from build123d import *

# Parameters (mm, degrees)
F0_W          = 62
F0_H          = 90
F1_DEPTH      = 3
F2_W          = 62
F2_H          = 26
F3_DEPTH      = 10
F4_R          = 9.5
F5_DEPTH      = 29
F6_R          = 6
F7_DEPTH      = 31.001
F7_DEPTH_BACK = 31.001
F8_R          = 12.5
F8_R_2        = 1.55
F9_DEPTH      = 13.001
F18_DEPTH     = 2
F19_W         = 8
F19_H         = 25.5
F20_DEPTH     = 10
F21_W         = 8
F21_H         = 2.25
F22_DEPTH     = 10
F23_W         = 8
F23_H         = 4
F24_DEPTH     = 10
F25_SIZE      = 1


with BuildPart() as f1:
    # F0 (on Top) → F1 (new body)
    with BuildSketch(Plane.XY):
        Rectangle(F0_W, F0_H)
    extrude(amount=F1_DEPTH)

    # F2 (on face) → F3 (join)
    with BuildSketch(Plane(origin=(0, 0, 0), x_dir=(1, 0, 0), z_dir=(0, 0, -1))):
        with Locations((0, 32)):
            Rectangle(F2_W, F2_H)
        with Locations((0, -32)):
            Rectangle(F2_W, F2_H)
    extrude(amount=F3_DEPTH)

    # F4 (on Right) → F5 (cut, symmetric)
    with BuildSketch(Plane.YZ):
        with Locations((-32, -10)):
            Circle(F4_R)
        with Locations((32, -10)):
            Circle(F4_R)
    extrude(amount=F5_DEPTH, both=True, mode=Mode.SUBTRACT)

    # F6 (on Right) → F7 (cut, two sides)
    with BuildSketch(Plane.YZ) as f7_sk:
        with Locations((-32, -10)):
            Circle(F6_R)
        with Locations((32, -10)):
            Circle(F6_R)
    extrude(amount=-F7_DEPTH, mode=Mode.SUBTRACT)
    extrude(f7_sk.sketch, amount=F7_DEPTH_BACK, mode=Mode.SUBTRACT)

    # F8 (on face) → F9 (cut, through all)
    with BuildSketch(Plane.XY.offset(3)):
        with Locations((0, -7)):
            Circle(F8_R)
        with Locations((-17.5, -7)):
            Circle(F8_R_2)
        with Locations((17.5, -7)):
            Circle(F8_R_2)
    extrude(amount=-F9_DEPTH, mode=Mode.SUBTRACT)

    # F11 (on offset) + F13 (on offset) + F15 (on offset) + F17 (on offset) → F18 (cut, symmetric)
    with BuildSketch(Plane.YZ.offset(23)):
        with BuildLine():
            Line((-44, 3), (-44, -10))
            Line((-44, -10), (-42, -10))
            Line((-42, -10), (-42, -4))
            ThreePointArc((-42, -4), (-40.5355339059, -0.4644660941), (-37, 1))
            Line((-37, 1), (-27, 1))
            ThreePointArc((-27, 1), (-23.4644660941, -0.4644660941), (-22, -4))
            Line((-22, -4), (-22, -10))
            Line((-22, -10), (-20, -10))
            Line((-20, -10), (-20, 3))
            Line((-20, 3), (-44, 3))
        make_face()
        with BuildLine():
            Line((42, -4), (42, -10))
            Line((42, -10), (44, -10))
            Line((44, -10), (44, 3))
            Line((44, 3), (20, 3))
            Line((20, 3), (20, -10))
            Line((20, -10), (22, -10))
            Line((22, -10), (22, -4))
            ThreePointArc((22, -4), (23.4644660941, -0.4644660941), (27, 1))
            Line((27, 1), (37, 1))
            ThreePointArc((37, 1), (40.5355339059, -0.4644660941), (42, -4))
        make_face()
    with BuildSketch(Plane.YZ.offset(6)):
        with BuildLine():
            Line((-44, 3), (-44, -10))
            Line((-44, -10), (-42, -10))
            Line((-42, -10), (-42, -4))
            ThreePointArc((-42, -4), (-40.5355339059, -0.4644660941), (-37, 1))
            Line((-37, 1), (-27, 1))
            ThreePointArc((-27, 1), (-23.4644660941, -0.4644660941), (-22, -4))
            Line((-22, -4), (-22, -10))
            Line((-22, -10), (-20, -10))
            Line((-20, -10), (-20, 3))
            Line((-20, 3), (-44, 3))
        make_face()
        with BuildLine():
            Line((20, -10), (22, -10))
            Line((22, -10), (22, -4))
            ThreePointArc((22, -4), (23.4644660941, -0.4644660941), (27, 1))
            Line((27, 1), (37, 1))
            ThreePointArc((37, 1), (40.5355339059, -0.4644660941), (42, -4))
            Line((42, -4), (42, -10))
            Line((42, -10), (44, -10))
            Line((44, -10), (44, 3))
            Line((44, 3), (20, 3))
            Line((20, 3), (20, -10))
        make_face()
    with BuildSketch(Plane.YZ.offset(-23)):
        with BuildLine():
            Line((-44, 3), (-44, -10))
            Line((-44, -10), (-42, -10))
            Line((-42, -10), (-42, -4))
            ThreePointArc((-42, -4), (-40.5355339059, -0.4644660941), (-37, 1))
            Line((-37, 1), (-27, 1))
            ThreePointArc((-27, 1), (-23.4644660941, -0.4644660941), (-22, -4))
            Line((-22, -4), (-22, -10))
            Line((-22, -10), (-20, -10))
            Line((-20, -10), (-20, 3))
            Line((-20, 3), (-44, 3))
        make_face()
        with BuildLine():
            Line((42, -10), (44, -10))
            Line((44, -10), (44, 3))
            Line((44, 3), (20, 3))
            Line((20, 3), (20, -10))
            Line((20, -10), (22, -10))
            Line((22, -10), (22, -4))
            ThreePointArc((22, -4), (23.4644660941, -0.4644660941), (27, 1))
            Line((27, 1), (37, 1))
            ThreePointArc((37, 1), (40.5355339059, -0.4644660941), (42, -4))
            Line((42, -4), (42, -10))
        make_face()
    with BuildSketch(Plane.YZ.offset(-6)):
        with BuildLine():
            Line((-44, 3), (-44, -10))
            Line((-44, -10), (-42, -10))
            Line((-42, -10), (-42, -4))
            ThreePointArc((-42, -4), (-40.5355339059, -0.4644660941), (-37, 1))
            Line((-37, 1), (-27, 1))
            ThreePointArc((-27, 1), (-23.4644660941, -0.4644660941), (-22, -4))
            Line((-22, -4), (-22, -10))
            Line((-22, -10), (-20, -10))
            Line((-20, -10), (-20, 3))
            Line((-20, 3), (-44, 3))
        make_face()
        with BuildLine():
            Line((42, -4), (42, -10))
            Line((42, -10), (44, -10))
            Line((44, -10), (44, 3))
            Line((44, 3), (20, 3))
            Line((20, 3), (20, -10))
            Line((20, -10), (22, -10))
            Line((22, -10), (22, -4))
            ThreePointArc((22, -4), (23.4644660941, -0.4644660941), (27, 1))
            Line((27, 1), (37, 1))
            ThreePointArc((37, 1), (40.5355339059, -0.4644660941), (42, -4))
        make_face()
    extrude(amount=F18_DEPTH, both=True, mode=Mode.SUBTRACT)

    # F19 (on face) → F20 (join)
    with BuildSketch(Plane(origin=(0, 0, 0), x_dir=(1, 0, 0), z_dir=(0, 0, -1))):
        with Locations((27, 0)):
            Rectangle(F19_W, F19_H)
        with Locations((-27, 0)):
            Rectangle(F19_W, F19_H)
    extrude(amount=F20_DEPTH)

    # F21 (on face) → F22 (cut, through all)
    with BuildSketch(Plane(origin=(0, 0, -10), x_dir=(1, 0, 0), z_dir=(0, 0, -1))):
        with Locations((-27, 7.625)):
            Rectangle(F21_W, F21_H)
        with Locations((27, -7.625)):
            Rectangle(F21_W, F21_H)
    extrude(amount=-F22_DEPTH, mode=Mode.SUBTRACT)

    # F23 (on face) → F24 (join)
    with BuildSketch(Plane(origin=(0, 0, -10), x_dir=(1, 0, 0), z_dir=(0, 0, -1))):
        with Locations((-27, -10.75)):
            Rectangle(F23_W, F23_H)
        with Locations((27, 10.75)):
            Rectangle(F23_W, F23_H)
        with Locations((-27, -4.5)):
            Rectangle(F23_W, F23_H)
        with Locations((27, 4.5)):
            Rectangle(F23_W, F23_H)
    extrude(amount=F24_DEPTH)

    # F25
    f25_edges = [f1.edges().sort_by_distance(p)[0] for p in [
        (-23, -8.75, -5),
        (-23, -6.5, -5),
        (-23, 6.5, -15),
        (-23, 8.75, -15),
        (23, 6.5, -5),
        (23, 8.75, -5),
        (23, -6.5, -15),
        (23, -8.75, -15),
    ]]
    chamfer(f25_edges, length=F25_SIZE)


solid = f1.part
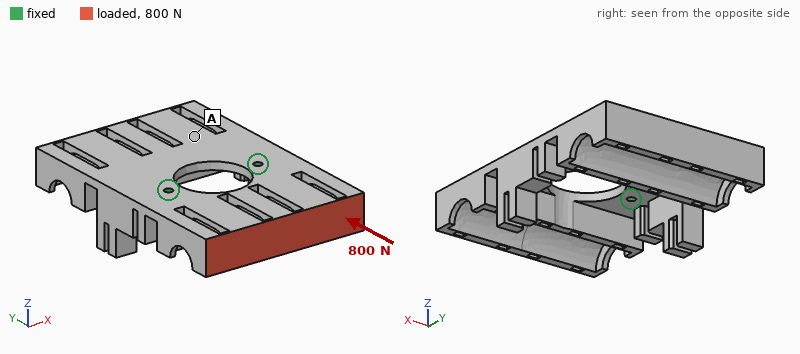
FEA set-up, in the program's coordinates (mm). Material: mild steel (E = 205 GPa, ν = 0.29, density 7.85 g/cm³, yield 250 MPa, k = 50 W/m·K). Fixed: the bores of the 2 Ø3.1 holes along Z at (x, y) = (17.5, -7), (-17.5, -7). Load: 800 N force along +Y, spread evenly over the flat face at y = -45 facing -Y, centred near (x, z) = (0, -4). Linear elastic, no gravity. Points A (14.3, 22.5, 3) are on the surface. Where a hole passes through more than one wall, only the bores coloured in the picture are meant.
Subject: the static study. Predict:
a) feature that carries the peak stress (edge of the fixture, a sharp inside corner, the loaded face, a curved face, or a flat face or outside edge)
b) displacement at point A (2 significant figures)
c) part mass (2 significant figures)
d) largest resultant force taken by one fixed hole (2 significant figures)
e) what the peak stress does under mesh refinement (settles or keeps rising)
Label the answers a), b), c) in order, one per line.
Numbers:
a) edge of the fixture
b) 0.015 mm
c) 250 g
d) 410 N
e) keeps rising
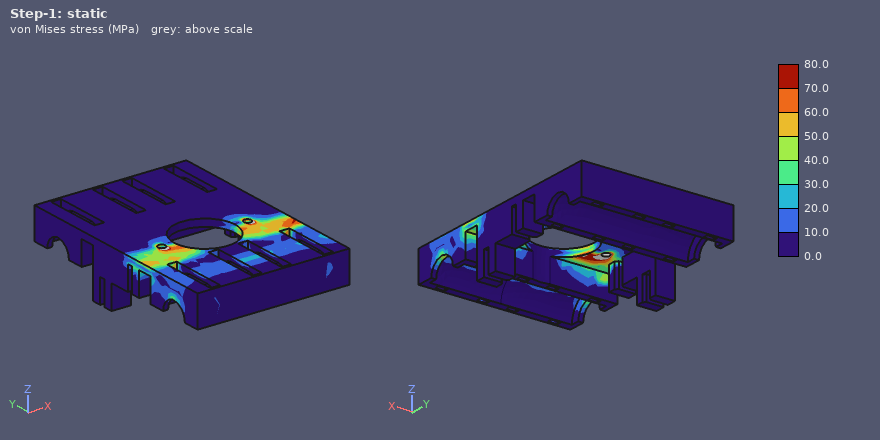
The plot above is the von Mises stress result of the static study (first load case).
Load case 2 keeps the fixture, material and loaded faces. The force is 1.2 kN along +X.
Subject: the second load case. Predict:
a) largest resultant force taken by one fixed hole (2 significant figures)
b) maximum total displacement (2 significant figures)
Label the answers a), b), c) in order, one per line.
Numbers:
a) 1.4 kN
b) 24 µm
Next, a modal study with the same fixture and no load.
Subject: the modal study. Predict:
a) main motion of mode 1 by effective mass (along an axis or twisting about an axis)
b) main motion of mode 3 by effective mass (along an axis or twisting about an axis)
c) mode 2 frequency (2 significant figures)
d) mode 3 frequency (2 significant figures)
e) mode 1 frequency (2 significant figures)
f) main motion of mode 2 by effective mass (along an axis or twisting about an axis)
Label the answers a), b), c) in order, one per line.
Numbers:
a) along Z
b) twisting about Y
c) 1000 Hz
d) 1700 Hz
e) 620 Hz
f) along Z
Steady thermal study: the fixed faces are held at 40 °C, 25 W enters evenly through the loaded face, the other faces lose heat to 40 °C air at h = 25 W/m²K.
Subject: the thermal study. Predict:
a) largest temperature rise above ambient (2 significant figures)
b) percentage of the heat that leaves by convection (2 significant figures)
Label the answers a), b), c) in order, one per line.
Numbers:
a) 80 K
b) 46 %
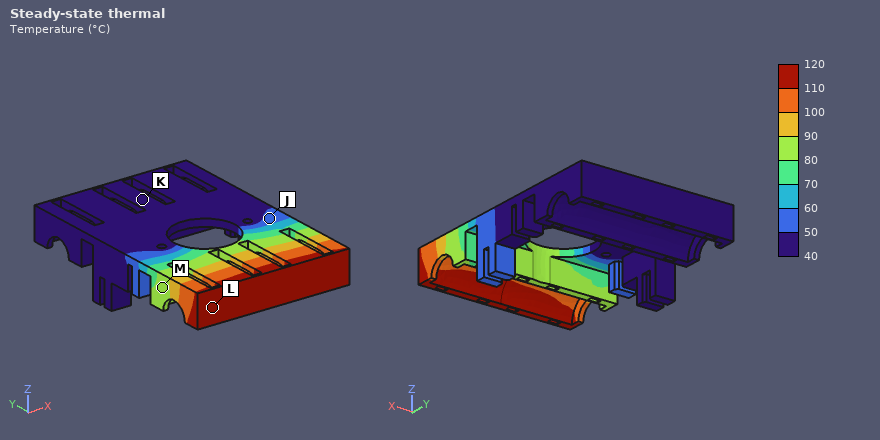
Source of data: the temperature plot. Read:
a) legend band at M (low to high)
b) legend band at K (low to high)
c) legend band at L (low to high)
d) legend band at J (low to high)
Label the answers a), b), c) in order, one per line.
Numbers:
a) 80 to 90 °C
b) 40 to 50 °C
c) 110 to 120 °C
d) 50 to 60 °C
